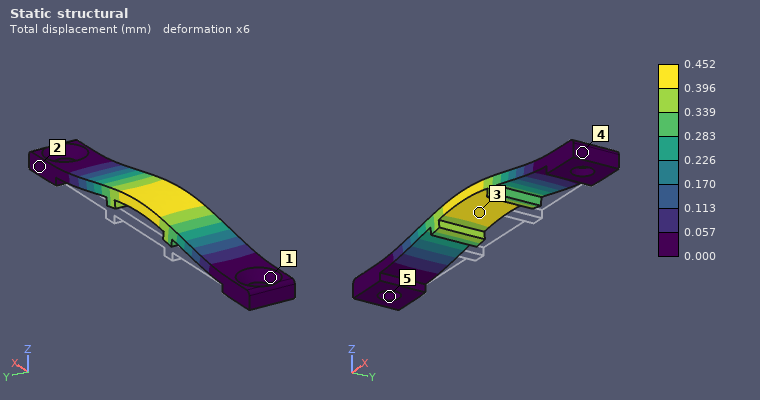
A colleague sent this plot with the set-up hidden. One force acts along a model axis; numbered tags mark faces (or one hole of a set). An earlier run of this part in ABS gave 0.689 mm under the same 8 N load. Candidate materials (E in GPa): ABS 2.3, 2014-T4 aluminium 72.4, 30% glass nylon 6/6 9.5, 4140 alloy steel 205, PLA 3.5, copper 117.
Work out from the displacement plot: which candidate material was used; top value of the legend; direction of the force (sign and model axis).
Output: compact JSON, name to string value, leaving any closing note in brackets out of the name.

{"which candidate material was used": "PLA", "top value of the legend": "0.452 mm", "direction of the force": "+Z"}
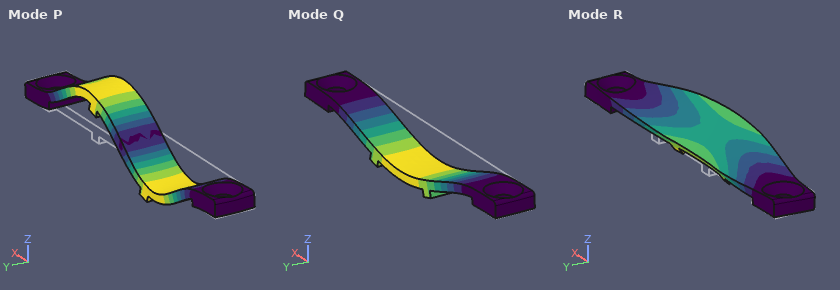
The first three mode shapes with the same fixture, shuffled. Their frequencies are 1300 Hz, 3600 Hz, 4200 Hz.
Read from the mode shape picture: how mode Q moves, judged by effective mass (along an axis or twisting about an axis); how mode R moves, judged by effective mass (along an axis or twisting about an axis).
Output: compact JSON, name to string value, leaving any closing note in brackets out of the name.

{"how mode Q moves, judged by effective mass": "along Z", "how mode R moves, judged by effective mass": "along Y"}
